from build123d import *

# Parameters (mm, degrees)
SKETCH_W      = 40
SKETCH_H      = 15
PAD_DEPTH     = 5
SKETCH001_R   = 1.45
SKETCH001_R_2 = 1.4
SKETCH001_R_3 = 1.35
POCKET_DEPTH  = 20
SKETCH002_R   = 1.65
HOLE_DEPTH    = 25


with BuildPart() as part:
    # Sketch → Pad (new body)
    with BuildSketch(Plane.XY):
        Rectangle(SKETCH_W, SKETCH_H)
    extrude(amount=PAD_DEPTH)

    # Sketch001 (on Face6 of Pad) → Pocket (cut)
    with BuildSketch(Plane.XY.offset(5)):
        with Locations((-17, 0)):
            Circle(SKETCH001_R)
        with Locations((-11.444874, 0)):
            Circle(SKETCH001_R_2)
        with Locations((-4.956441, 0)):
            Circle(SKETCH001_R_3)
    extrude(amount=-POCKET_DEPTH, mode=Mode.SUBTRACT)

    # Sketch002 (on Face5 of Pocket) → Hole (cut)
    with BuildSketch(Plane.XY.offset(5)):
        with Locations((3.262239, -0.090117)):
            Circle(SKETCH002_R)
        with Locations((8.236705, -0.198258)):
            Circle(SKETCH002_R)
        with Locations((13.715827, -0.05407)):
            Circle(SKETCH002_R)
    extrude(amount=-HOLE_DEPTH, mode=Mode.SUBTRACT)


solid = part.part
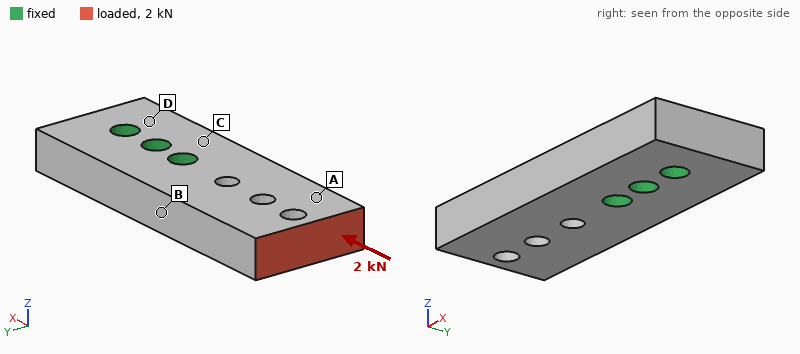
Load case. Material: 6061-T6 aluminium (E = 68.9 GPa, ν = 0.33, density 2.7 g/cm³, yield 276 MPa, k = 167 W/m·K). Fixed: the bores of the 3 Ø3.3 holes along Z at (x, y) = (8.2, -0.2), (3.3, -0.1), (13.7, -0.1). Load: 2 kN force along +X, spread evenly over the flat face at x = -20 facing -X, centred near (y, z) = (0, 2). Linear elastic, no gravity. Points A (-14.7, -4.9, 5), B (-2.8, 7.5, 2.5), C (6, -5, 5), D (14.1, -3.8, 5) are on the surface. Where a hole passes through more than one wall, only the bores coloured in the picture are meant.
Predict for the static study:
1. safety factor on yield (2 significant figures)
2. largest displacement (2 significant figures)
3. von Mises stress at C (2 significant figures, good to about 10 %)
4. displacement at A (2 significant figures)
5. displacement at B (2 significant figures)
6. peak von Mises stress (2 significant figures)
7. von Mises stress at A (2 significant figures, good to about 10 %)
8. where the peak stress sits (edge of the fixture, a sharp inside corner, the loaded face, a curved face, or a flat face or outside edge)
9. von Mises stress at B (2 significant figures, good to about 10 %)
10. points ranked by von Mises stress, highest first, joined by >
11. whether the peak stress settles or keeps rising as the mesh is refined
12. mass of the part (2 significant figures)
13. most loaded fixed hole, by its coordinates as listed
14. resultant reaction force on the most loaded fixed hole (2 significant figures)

3.0
13 µm
13 MPa
8.7 µm
4.1 µm
93 MPa
32 MPa
a curved face
22 MPa
A > B > C > D
settles
7.5 g
(3.3, -0.1)
1.4 kN
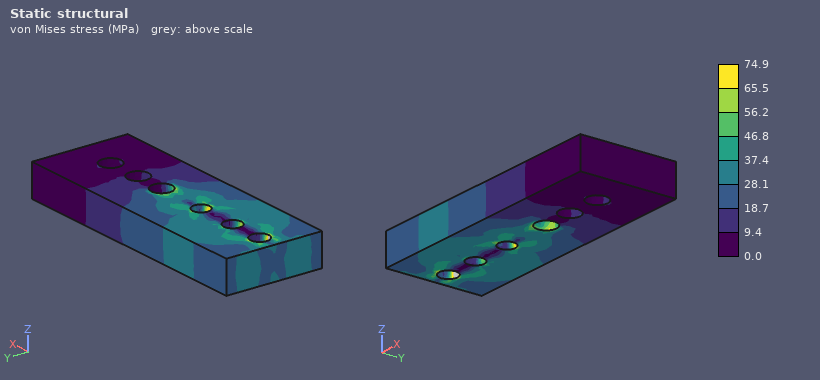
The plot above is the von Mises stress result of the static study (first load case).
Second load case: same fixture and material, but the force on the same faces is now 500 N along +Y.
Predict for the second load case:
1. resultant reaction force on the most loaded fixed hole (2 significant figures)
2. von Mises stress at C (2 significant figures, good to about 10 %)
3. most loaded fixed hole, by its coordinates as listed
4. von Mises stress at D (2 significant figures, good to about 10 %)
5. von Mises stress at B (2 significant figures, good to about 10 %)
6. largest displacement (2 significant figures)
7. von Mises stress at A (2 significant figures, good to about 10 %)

1.3 kN
32 MPa
(3.3, -0.1)
8.9 MPa
51 MPa
51 µm
12 MPa
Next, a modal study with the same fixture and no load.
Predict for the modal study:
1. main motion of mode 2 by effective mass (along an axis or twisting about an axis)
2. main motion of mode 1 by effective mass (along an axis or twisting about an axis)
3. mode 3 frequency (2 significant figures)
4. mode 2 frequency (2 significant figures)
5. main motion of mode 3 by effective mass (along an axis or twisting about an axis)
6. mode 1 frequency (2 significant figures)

along Y
along Z
18 kHz
14 kHz
twisting about X
7400 Hz
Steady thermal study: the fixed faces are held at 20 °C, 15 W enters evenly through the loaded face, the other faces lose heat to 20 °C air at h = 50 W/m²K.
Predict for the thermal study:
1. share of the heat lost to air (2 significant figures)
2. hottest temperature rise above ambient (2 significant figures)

5.3 %
31 K
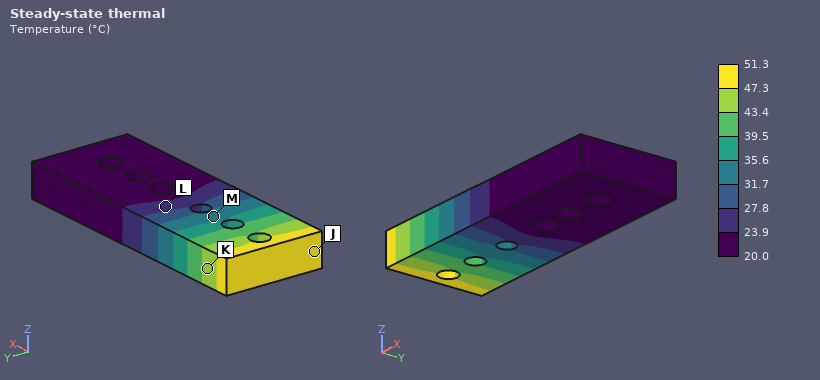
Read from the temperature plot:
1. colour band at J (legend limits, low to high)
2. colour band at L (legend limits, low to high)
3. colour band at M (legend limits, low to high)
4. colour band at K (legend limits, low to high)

47.3 to 51.3 °C
23.9 to 27.8 °C
31.7 to 35.6 °C
43.4 to 47.3 °C
